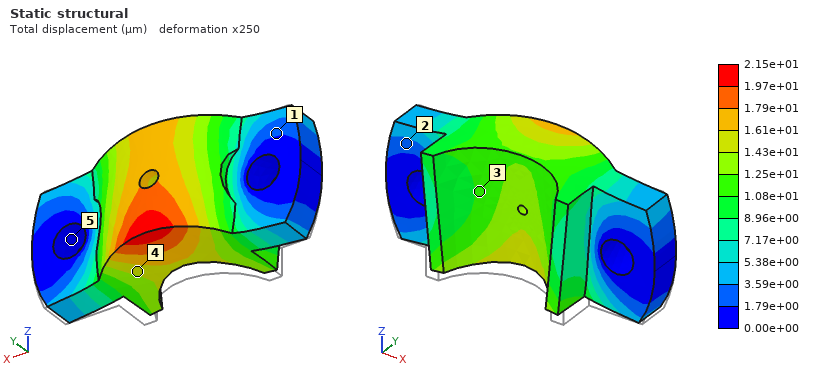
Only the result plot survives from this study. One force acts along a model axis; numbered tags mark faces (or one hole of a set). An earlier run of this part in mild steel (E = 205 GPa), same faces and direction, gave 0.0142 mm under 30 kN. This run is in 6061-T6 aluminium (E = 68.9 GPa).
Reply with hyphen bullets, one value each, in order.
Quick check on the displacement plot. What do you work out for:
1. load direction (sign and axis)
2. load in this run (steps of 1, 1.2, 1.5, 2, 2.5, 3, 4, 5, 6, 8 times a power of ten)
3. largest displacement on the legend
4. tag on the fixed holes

- +Z
- 15 kN
- 2.15e+01 µm
- 5
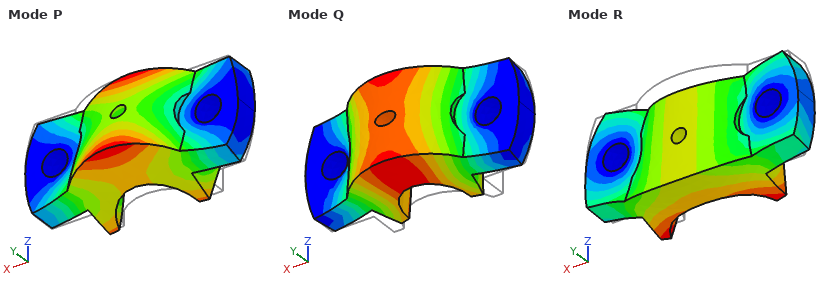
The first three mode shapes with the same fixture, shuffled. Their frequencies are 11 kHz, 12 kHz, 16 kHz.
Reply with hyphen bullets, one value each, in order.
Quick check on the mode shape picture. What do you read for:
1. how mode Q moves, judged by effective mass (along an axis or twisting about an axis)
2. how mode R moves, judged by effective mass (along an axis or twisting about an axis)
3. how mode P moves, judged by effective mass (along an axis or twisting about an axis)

- along Y
- along Z
- twisting about X
